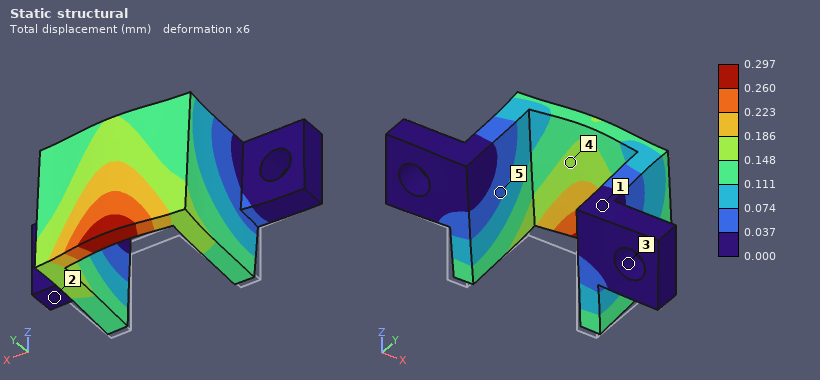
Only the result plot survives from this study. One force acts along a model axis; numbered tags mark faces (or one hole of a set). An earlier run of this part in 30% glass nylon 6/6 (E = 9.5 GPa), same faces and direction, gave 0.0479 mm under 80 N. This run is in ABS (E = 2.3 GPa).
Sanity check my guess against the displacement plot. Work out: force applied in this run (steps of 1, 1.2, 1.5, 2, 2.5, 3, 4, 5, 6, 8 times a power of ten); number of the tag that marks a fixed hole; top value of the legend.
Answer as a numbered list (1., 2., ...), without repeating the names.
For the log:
1. 120 N
2. 3
3. 0.297 mm
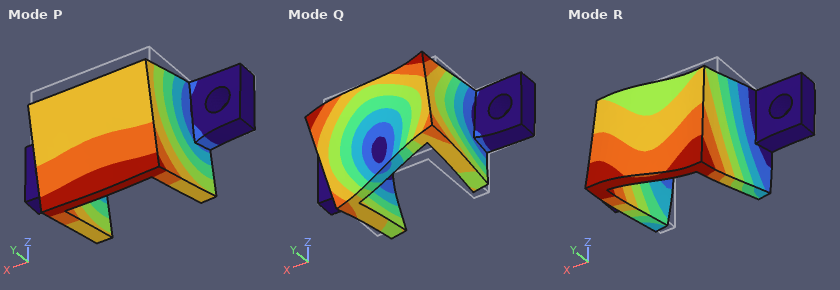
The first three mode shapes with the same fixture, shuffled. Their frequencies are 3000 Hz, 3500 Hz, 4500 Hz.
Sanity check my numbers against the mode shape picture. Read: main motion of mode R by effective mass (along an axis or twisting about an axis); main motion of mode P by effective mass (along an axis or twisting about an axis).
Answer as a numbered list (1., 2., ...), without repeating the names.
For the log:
1. along X
2. along Z
